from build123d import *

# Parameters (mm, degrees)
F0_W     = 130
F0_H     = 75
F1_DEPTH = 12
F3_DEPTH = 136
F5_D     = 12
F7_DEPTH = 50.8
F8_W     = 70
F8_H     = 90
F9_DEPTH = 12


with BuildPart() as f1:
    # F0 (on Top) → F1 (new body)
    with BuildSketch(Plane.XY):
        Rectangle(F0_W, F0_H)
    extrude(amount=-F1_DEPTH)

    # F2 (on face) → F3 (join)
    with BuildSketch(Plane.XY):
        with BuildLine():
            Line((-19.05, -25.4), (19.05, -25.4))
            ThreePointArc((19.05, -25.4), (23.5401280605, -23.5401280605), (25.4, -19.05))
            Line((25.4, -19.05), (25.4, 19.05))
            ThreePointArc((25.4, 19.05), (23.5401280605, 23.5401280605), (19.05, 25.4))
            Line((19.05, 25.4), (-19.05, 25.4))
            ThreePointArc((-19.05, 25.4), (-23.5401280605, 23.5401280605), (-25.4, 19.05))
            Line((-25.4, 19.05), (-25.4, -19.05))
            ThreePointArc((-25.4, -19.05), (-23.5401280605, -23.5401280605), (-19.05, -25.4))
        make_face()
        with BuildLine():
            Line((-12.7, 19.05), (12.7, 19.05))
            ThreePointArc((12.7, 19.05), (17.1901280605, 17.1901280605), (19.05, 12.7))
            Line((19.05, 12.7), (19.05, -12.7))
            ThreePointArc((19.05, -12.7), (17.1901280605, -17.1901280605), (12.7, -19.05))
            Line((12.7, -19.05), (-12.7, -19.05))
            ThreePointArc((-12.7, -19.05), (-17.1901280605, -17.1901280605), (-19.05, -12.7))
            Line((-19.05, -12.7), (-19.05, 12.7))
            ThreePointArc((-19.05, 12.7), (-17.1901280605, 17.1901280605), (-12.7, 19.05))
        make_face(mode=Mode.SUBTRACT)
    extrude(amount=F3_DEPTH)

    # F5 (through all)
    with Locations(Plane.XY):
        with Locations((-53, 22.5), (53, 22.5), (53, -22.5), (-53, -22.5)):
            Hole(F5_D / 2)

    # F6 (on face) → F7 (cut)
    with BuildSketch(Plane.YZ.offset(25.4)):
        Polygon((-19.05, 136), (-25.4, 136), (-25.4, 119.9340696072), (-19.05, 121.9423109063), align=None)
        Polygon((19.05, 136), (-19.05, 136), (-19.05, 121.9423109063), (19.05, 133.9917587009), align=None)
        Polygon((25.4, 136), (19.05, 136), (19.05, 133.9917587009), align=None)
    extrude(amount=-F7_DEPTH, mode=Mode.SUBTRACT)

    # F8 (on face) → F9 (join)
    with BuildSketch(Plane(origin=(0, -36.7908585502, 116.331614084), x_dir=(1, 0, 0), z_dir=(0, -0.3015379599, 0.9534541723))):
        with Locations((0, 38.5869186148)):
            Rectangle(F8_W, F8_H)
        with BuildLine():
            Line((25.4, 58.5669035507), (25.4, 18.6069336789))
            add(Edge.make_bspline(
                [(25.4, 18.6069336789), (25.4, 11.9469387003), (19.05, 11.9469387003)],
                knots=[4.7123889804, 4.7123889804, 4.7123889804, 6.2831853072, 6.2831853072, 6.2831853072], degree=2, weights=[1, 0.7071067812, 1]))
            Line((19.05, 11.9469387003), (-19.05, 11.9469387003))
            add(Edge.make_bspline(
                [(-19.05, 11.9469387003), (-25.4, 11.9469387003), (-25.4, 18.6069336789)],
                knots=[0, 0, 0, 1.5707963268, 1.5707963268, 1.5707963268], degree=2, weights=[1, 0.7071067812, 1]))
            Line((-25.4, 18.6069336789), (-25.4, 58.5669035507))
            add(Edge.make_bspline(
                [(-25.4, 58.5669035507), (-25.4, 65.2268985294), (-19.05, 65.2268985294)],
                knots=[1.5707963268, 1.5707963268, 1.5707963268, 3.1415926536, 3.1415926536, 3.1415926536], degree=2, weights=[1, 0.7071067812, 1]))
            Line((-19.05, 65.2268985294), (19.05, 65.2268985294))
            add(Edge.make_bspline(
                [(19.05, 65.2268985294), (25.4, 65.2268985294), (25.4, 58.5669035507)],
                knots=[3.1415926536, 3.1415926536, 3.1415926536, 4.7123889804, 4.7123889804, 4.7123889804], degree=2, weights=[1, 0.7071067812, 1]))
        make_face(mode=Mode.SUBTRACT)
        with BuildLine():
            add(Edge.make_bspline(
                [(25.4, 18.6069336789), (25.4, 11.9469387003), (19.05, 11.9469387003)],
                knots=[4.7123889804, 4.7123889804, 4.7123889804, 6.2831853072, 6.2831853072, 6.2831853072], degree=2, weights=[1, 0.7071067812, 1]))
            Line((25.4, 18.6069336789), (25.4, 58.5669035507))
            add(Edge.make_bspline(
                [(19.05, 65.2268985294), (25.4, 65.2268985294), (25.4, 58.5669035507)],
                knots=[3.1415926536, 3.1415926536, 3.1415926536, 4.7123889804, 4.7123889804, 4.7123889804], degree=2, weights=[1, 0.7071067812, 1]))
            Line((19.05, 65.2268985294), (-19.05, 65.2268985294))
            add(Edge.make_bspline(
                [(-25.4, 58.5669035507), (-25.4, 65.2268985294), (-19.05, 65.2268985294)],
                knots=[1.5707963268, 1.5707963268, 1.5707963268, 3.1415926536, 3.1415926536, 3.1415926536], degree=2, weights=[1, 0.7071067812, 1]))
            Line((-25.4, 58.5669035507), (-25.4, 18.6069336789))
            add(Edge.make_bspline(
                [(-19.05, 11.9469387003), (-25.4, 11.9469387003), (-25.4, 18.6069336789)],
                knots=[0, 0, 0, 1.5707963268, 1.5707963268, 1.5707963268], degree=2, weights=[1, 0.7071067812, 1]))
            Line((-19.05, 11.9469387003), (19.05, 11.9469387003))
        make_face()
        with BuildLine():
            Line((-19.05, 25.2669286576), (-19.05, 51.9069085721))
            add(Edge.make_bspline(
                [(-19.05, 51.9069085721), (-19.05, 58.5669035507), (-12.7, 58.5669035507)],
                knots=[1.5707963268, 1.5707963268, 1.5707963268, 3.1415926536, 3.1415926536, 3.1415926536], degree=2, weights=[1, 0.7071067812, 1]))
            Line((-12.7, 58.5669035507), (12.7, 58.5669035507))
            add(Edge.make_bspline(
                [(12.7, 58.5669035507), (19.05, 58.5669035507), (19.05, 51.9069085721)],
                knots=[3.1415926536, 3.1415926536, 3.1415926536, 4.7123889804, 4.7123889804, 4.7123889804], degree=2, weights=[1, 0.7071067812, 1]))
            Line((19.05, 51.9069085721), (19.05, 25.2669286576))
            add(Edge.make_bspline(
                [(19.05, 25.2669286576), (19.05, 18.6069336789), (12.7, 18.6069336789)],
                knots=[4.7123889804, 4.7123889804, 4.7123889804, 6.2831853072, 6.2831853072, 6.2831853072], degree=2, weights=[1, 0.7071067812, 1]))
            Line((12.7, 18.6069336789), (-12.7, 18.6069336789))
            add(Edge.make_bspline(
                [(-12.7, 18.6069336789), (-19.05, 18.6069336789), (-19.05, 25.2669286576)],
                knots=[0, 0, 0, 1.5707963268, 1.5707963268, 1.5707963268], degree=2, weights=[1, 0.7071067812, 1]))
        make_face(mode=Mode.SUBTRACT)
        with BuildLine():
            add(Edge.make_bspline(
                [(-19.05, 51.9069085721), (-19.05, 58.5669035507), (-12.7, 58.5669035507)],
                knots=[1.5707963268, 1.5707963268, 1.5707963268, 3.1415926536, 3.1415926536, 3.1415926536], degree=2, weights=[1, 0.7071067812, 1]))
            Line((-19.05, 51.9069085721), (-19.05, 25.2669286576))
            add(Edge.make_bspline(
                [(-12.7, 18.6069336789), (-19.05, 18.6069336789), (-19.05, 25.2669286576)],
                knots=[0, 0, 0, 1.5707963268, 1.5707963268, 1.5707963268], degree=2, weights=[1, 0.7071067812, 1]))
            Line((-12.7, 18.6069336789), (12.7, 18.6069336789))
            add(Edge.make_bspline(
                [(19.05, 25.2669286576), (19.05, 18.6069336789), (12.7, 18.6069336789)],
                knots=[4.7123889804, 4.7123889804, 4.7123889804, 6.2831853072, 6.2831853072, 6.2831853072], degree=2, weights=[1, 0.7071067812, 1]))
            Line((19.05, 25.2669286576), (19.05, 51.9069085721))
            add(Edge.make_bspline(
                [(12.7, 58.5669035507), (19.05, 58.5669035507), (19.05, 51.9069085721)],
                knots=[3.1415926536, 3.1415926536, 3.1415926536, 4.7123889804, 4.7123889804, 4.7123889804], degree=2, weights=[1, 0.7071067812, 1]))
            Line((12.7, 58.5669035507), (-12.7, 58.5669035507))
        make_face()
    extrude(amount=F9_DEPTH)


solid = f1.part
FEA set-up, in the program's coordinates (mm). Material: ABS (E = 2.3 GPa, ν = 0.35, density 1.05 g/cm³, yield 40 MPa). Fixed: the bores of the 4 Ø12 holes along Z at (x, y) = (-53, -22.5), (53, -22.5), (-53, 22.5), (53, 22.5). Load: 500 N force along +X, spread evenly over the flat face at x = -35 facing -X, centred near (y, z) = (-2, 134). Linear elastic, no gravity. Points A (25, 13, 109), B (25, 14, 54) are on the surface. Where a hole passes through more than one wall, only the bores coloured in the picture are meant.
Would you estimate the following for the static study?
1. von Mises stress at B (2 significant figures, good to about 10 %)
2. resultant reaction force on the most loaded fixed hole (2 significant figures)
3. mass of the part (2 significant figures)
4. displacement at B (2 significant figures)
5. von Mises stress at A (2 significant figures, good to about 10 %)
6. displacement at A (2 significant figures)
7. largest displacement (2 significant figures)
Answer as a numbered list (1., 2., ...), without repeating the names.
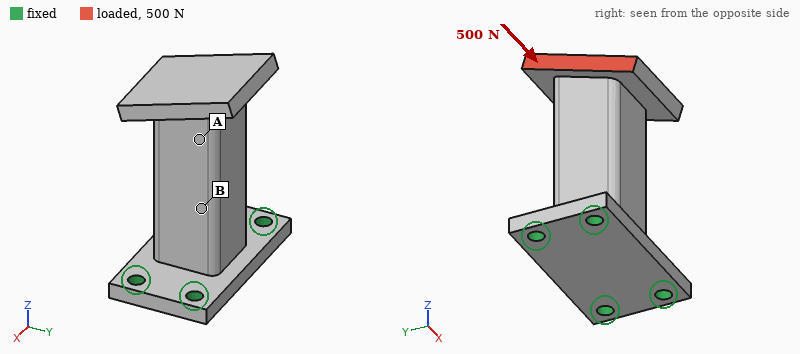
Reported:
1. 2.8 MPa
2. 480 N
3. 350 g
4. 0.44 mm
5. 1.0 MPa
6. 0.96 mm
7. 1.4 mm
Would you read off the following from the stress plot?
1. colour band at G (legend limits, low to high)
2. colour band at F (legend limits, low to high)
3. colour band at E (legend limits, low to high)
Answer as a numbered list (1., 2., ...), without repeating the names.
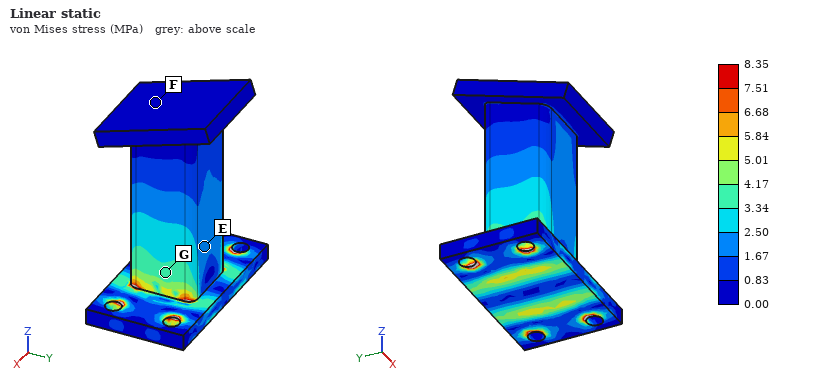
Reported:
1. 3.34 to 4.17 MPa
2. 0.00 to 0.83 MPa
3. 1.67 to 2.50 MPa
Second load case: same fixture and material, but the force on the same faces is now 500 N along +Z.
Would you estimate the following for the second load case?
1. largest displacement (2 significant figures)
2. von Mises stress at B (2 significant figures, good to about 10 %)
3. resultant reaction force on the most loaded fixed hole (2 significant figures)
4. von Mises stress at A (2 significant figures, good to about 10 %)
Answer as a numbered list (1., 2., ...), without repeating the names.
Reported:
1. 0.51 mm
2. 0.80 MPa
3. 250 N
4. 0.69 MPa
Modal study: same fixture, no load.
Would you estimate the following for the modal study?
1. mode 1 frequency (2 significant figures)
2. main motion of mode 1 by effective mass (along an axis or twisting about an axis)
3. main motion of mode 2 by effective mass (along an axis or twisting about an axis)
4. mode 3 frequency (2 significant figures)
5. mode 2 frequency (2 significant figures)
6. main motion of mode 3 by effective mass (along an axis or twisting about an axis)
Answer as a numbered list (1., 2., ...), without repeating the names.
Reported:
1. 210 Hz
2. along Y
3. along X
4. 880 Hz
5. 290 Hz
6. along Z
